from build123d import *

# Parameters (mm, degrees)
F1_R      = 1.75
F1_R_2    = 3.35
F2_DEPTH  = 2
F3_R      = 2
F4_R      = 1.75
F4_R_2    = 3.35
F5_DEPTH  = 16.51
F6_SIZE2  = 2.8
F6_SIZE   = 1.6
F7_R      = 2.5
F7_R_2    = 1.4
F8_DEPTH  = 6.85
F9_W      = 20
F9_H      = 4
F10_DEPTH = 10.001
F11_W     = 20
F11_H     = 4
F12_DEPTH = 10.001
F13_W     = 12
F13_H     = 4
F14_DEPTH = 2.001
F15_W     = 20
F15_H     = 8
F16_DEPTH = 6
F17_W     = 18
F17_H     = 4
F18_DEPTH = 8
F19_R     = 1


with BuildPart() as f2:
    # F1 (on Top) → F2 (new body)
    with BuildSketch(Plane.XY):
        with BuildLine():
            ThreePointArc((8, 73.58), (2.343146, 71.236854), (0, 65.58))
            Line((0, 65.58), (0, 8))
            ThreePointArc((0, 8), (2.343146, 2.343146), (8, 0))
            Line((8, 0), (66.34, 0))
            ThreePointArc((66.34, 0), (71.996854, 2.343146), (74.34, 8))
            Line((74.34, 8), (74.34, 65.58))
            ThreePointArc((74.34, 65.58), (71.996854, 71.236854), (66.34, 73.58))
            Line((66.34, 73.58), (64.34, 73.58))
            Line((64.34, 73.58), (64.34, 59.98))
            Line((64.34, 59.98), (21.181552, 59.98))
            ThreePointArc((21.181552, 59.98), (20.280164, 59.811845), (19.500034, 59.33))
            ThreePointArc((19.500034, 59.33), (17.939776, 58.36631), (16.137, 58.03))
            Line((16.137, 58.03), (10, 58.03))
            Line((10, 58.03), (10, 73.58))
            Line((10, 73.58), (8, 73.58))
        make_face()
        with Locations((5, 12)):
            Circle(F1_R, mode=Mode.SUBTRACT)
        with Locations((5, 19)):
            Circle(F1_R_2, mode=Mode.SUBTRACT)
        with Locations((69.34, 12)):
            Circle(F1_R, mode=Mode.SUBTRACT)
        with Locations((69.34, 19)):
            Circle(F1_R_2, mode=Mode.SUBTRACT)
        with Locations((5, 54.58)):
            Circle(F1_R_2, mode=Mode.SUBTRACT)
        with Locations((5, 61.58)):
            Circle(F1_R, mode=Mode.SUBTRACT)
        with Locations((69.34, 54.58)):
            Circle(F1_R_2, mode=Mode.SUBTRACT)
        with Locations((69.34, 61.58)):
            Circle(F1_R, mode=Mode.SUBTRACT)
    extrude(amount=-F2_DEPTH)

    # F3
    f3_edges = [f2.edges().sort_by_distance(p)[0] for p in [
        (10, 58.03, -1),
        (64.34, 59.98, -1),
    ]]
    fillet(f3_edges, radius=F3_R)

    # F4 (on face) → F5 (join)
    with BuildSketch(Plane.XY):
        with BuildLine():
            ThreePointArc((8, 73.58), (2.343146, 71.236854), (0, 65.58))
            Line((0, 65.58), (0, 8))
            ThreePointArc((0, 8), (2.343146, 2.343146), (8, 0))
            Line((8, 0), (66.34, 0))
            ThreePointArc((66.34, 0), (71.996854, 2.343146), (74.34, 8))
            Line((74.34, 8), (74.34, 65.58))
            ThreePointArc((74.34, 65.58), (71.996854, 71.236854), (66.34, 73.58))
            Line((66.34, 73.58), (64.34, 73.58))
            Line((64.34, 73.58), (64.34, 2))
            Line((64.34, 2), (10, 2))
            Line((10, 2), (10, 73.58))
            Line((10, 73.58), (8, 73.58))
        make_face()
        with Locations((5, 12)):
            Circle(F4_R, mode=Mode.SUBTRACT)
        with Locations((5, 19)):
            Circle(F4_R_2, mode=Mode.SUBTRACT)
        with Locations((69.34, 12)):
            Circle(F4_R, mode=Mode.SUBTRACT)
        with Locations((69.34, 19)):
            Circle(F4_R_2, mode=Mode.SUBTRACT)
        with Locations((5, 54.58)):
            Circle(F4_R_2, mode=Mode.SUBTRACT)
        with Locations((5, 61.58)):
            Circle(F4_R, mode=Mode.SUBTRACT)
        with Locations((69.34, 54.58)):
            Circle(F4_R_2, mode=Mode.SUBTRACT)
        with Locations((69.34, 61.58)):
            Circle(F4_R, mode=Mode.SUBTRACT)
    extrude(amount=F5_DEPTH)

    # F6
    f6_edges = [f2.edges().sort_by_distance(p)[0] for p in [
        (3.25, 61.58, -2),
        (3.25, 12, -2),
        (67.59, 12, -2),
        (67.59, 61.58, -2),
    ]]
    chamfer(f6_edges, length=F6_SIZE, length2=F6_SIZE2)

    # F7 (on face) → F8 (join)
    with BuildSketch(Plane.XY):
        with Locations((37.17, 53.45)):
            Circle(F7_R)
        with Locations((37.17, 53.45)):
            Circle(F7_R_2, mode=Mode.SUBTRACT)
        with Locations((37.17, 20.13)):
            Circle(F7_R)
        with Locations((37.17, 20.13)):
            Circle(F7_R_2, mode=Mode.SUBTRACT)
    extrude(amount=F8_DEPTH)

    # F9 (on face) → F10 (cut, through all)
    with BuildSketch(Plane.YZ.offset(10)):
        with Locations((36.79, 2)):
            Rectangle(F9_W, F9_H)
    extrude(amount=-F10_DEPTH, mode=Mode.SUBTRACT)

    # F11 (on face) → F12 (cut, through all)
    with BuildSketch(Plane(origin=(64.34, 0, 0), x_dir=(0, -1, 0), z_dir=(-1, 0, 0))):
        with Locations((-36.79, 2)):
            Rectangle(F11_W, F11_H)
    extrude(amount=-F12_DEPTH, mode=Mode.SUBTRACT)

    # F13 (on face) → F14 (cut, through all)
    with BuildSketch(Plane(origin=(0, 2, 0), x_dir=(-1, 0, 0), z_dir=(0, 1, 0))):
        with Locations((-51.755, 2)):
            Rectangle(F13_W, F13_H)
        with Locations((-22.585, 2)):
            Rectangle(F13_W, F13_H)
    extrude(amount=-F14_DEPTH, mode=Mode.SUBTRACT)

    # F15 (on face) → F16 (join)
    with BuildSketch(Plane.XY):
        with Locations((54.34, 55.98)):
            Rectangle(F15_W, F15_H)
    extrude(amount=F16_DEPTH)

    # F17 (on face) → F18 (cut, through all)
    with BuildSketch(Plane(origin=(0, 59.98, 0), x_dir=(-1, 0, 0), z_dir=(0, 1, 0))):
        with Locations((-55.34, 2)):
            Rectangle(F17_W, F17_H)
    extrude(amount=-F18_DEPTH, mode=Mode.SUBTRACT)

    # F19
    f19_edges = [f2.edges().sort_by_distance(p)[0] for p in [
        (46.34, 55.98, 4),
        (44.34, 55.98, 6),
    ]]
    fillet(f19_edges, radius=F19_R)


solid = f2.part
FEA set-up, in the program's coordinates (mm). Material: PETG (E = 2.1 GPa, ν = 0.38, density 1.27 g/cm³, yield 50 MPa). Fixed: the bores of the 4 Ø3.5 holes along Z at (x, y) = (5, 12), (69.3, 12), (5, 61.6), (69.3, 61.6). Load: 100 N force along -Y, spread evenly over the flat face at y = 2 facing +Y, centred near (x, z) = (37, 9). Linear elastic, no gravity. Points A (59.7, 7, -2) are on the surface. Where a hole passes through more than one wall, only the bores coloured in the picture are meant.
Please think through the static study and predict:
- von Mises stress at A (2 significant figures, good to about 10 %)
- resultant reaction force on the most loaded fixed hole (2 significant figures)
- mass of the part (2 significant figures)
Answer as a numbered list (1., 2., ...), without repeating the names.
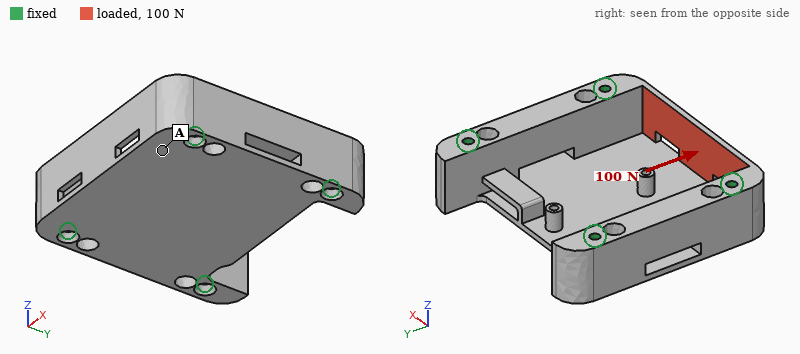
1. 1.7 MPa
2. 42 N
3. 38 g
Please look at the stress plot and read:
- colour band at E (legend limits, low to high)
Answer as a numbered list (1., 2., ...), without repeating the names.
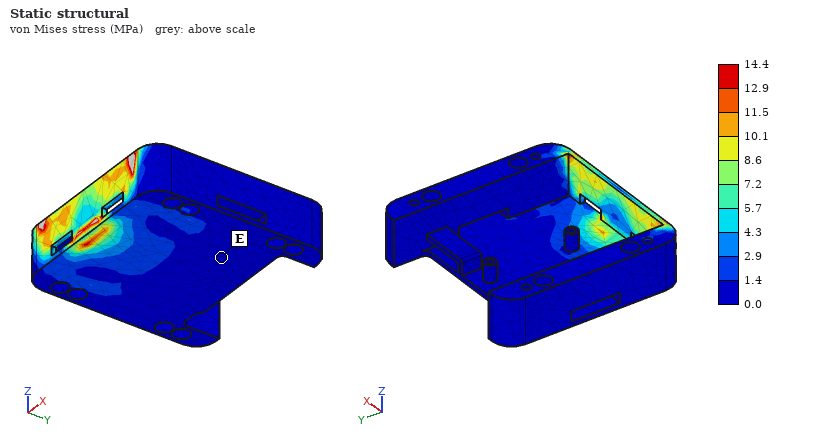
1. 0.0 to 1.4 MPa
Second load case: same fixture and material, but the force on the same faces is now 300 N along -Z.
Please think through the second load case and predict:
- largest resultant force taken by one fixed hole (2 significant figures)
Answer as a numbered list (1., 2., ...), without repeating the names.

1. 150 N
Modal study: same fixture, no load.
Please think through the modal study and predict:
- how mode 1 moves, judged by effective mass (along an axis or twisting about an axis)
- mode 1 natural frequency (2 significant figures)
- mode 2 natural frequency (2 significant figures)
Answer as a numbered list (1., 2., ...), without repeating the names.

1. along Z
2. 910 Hz
3. 1300 Hz
